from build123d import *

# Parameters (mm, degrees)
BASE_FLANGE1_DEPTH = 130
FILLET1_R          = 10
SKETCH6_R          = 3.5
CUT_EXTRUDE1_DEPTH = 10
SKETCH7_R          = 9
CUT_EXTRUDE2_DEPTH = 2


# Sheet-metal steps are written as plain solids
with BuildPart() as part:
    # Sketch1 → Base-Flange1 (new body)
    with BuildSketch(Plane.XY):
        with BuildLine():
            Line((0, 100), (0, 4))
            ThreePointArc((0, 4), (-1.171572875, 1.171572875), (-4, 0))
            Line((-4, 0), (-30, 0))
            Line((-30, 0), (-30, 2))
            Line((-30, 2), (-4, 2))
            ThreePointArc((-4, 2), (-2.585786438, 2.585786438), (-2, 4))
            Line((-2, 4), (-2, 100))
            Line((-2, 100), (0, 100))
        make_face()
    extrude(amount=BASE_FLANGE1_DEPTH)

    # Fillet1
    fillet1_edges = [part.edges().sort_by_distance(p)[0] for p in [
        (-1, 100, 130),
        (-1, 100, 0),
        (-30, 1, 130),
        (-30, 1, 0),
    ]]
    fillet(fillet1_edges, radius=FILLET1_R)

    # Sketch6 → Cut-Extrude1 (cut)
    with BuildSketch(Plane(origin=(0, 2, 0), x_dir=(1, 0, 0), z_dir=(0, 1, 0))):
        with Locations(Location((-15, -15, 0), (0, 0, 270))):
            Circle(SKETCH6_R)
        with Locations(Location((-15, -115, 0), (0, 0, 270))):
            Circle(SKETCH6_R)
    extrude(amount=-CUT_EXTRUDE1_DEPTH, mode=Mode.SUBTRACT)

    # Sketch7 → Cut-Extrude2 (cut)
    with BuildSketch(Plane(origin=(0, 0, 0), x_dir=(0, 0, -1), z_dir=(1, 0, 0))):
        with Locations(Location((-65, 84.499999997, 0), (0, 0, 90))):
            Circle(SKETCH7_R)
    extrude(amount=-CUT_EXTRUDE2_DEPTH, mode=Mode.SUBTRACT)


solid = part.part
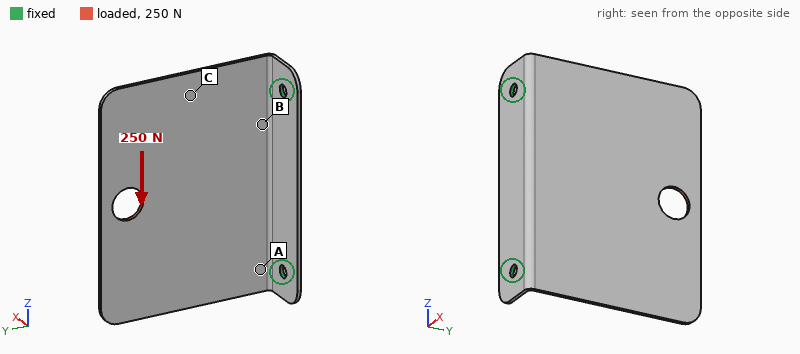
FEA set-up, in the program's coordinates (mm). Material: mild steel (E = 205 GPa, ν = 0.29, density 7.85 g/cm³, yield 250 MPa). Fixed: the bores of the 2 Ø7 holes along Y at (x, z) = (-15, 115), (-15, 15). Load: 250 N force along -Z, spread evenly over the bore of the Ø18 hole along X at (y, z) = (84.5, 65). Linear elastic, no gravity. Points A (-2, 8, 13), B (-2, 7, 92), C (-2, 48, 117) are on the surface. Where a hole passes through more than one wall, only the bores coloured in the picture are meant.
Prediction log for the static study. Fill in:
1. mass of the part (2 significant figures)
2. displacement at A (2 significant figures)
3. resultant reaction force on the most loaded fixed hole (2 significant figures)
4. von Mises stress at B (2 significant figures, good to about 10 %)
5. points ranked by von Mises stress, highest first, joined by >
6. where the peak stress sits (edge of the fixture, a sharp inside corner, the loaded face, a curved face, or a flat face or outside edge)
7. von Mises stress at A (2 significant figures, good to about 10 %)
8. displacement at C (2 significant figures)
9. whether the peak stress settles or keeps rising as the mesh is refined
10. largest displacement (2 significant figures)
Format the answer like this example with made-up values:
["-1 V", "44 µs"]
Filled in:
["250 g", "0.028 mm", "240 N", "14 MPa", "A > B > C", "edge of the fixture", "24 MPa", "0.070 mm", "keeps rising", "0.11 mm"]
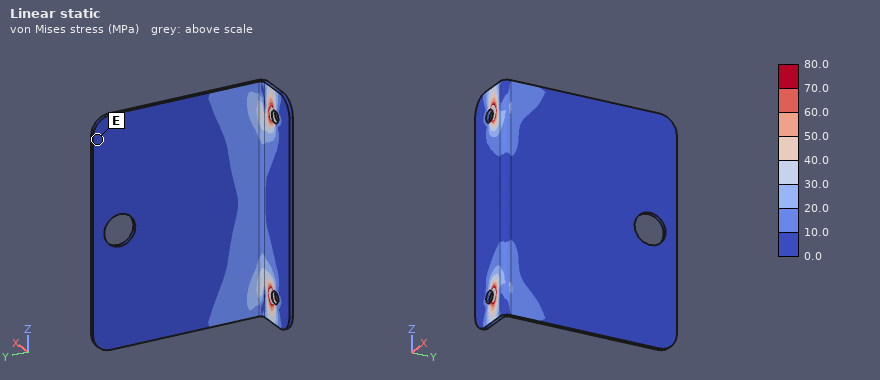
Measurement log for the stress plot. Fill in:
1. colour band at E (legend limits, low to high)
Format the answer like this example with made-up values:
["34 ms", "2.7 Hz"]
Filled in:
["0.0 to 10.0 MPa"]
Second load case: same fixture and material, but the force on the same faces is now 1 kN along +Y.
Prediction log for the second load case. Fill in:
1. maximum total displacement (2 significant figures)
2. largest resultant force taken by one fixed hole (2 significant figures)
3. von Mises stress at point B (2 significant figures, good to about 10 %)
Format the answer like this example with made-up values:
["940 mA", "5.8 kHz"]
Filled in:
["0.67 mm", "510 N", "18 MPa"]
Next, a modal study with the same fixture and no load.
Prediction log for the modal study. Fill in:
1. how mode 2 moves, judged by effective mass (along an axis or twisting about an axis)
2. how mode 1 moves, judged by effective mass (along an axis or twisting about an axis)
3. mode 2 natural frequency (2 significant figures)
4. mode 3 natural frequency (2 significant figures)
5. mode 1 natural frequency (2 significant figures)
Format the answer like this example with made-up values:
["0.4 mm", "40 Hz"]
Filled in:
["twisting about Y", "along X", "310 Hz", "820 Hz", "130 Hz"]
